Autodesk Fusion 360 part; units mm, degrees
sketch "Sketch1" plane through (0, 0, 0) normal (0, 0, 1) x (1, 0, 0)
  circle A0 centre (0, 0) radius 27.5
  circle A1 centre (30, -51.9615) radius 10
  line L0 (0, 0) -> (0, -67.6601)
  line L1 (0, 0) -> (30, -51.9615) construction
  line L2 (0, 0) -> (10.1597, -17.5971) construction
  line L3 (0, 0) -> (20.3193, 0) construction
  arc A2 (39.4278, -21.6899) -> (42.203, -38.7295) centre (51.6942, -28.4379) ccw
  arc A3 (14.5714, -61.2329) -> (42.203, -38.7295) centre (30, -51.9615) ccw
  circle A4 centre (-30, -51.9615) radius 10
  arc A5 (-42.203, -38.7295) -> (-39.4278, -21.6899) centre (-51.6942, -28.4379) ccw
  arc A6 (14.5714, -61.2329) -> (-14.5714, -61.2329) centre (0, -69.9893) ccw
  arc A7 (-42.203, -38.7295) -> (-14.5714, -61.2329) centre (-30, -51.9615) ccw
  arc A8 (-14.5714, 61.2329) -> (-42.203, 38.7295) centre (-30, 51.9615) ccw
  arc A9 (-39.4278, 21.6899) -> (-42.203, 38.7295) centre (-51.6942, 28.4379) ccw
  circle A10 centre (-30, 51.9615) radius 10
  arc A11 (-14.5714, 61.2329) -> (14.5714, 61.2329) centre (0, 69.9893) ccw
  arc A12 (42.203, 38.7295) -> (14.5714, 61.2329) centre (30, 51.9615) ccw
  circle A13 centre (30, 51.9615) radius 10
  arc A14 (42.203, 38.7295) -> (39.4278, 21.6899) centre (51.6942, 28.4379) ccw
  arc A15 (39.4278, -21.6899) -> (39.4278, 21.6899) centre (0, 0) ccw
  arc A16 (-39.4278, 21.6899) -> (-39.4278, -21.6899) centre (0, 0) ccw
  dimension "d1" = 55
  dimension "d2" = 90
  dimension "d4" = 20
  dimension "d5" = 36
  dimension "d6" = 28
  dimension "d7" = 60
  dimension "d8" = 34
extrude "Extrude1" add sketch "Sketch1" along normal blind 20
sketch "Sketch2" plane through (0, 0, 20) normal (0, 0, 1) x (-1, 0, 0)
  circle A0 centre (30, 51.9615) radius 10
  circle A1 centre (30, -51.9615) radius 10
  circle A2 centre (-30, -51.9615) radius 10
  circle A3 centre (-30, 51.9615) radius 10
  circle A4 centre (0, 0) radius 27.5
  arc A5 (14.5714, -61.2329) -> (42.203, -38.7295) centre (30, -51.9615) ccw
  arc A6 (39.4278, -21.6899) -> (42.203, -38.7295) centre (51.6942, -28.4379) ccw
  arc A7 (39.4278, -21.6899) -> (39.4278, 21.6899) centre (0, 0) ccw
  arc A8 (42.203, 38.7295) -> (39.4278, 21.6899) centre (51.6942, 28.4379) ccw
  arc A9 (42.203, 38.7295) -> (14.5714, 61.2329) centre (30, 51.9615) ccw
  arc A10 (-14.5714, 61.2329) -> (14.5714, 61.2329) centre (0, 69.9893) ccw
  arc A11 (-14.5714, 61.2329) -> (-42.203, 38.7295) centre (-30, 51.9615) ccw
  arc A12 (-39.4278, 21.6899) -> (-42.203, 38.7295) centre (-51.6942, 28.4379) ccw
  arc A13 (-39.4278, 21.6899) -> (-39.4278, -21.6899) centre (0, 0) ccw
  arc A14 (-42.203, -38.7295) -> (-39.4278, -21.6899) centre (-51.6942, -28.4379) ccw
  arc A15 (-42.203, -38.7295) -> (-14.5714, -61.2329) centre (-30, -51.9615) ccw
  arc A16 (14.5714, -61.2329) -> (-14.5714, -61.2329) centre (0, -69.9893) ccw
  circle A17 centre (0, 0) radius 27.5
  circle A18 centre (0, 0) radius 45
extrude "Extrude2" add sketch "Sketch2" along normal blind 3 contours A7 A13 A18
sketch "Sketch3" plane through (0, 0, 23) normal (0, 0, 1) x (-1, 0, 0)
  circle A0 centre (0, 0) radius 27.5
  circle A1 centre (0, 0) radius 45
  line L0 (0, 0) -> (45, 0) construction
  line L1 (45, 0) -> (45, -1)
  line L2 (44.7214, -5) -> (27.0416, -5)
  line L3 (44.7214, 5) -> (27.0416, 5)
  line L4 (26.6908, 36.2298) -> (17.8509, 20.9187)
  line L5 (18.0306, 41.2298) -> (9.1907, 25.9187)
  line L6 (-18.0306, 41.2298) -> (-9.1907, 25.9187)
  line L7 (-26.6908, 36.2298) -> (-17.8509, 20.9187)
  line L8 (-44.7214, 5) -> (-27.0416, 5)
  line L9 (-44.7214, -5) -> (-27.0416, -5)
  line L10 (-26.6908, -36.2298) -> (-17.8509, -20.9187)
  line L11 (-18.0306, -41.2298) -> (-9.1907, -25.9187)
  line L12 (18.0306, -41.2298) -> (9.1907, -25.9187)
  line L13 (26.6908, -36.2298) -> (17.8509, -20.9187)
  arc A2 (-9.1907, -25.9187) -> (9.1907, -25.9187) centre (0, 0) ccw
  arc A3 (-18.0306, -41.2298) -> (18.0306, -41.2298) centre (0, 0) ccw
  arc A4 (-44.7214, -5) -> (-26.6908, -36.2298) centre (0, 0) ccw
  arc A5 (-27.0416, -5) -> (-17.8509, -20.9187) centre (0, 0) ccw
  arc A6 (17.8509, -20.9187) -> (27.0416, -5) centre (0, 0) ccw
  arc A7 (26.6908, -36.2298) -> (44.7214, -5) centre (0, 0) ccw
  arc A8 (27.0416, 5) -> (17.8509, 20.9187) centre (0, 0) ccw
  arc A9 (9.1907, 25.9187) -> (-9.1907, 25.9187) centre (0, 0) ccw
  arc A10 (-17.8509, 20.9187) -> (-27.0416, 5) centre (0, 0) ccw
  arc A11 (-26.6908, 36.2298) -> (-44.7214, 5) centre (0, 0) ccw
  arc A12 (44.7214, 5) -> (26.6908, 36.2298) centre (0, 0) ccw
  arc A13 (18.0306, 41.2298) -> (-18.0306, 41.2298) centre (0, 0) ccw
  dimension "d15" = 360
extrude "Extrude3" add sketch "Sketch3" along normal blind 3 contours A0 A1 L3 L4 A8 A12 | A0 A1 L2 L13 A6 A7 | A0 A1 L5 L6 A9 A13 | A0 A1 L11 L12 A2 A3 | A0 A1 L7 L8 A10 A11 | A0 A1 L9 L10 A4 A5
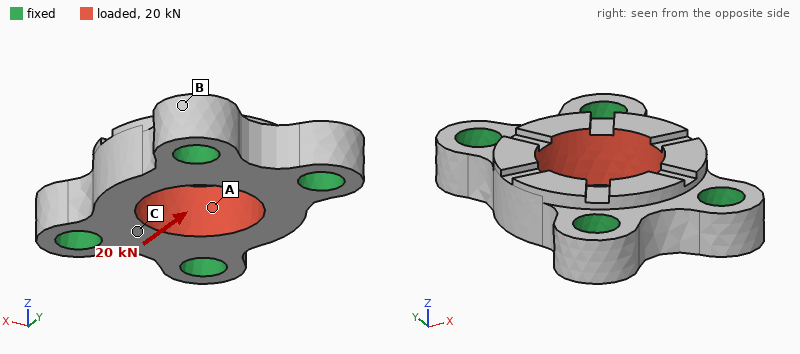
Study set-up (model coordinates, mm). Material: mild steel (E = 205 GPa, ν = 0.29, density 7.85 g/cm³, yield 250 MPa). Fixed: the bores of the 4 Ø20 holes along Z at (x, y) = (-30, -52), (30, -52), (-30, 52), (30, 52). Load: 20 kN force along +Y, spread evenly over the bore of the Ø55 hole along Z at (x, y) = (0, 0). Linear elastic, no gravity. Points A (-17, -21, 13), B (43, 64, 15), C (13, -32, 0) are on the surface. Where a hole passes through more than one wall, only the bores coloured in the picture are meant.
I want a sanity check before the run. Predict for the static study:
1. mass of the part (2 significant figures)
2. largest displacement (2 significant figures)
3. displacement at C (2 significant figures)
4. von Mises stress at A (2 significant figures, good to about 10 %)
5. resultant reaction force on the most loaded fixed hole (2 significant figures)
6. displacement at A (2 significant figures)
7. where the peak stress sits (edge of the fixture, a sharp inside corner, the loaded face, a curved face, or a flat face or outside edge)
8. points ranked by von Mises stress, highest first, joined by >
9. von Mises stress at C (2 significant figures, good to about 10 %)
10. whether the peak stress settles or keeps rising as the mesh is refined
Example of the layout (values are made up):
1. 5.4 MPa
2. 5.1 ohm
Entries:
1. 1.3 kg
2. 1.5 µm
3. 0.63 µm
4. 7.1 MPa
5. 5.2 kN
6. 0.99 µm
7. edge of the fixture
8. A > C > B
9. 4.3 MPa
10. keeps rising
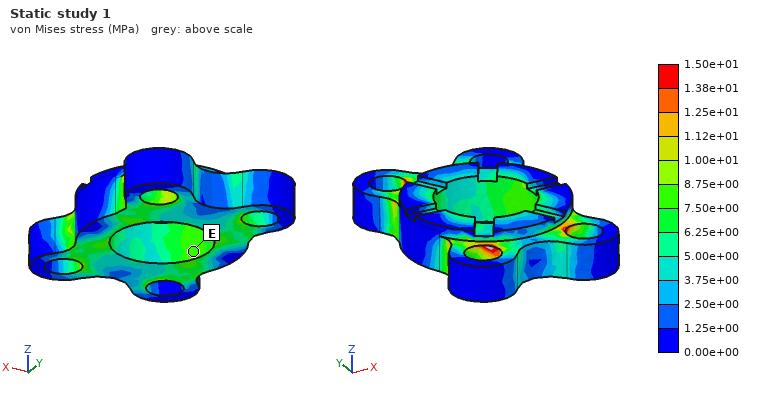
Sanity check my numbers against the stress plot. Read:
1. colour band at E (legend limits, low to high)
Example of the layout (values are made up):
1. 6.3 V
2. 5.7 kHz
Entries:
1. 7.50e+00 to 8.75e+00 MPa
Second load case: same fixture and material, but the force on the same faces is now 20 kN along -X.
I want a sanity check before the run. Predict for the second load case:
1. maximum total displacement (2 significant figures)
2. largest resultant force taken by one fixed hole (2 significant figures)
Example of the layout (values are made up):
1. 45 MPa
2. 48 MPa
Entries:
1. 4.5 µm
2. 5.3 kN
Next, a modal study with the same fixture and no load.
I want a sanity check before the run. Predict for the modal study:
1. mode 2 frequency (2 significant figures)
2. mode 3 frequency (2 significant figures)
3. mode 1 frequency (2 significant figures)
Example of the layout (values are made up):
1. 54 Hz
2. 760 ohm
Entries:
1. 11 kHz
2. 16 kHz
3. 10 kHz
